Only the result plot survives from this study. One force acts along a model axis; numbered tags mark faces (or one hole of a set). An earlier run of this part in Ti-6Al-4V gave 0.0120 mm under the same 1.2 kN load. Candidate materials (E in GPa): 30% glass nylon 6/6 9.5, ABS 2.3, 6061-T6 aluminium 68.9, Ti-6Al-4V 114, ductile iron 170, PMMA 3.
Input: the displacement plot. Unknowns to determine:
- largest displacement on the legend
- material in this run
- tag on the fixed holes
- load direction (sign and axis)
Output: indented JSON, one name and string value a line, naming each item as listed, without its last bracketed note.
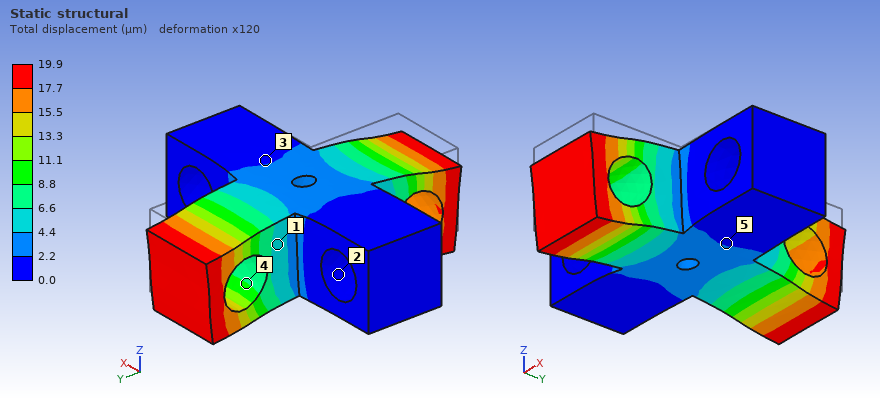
{
  "largest displacement on the legend": "19.9 µm",
  "material in this run": "6061-T6 aluminium",
  "tag on the fixed holes": "2",
  "load direction": "-Z"
}
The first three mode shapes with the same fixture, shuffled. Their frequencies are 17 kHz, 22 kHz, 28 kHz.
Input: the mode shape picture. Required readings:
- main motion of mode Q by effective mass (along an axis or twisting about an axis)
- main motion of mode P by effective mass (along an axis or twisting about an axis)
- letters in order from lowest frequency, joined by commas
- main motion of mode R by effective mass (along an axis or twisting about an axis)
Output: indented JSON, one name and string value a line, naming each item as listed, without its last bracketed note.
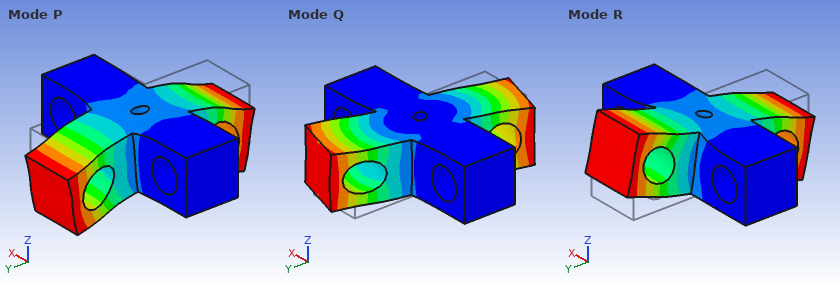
{
  "main motion of mode Q by effective mass": "twisting about Z",
  "main motion of mode P by effective mass": "along Z",
  "letters in order from lowest frequency, joined by commas": "R, P, Q",
  "main motion of mode R by effective mass": "twisting about X"
}
